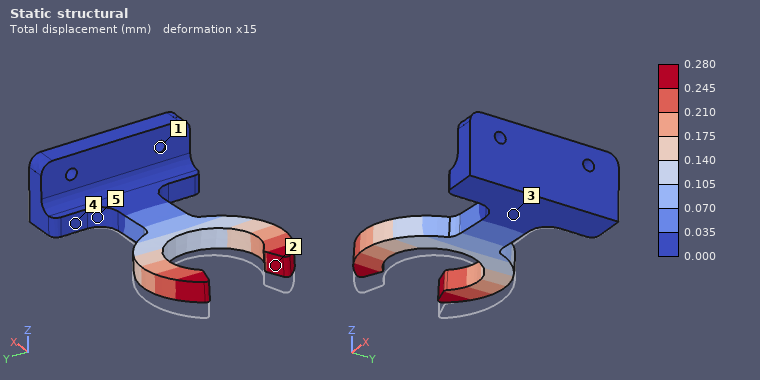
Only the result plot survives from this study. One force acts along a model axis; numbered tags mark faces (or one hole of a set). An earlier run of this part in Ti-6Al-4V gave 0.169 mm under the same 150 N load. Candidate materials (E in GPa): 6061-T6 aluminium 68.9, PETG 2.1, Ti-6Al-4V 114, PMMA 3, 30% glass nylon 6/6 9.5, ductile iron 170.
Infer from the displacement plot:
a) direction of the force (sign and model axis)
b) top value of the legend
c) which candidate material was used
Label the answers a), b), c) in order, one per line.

a) +Z
b) 0.280 mm
c) 6061-T6 aluminium
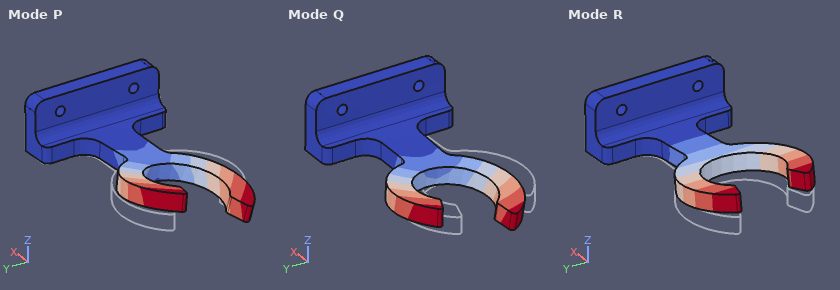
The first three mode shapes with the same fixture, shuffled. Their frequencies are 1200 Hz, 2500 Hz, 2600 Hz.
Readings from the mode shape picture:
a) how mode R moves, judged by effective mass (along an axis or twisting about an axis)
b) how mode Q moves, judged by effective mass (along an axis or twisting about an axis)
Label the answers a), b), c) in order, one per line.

a) along Z
b) along Y
